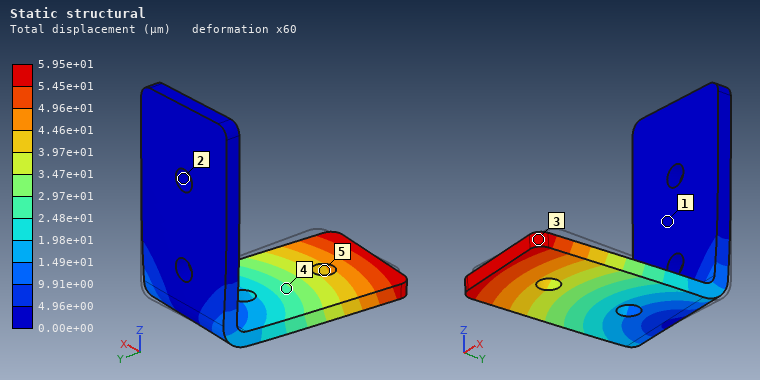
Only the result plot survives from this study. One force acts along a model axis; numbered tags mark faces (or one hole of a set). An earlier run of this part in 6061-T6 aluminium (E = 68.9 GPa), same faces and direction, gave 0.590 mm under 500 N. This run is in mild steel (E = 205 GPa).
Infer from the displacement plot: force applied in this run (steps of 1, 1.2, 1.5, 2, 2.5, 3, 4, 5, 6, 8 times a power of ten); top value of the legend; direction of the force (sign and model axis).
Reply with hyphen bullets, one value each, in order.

- 150 N
- 5.95e+01 µm
- -X
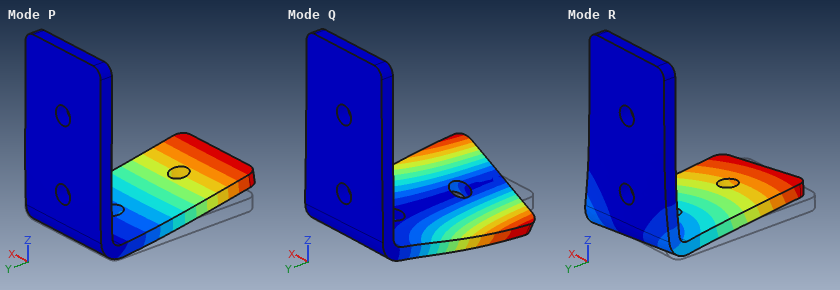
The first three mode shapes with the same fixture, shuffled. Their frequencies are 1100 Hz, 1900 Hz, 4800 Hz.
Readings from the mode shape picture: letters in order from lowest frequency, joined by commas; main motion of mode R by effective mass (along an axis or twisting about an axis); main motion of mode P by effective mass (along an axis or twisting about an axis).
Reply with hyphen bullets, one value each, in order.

- P, R, Q
- along X
- along Z
